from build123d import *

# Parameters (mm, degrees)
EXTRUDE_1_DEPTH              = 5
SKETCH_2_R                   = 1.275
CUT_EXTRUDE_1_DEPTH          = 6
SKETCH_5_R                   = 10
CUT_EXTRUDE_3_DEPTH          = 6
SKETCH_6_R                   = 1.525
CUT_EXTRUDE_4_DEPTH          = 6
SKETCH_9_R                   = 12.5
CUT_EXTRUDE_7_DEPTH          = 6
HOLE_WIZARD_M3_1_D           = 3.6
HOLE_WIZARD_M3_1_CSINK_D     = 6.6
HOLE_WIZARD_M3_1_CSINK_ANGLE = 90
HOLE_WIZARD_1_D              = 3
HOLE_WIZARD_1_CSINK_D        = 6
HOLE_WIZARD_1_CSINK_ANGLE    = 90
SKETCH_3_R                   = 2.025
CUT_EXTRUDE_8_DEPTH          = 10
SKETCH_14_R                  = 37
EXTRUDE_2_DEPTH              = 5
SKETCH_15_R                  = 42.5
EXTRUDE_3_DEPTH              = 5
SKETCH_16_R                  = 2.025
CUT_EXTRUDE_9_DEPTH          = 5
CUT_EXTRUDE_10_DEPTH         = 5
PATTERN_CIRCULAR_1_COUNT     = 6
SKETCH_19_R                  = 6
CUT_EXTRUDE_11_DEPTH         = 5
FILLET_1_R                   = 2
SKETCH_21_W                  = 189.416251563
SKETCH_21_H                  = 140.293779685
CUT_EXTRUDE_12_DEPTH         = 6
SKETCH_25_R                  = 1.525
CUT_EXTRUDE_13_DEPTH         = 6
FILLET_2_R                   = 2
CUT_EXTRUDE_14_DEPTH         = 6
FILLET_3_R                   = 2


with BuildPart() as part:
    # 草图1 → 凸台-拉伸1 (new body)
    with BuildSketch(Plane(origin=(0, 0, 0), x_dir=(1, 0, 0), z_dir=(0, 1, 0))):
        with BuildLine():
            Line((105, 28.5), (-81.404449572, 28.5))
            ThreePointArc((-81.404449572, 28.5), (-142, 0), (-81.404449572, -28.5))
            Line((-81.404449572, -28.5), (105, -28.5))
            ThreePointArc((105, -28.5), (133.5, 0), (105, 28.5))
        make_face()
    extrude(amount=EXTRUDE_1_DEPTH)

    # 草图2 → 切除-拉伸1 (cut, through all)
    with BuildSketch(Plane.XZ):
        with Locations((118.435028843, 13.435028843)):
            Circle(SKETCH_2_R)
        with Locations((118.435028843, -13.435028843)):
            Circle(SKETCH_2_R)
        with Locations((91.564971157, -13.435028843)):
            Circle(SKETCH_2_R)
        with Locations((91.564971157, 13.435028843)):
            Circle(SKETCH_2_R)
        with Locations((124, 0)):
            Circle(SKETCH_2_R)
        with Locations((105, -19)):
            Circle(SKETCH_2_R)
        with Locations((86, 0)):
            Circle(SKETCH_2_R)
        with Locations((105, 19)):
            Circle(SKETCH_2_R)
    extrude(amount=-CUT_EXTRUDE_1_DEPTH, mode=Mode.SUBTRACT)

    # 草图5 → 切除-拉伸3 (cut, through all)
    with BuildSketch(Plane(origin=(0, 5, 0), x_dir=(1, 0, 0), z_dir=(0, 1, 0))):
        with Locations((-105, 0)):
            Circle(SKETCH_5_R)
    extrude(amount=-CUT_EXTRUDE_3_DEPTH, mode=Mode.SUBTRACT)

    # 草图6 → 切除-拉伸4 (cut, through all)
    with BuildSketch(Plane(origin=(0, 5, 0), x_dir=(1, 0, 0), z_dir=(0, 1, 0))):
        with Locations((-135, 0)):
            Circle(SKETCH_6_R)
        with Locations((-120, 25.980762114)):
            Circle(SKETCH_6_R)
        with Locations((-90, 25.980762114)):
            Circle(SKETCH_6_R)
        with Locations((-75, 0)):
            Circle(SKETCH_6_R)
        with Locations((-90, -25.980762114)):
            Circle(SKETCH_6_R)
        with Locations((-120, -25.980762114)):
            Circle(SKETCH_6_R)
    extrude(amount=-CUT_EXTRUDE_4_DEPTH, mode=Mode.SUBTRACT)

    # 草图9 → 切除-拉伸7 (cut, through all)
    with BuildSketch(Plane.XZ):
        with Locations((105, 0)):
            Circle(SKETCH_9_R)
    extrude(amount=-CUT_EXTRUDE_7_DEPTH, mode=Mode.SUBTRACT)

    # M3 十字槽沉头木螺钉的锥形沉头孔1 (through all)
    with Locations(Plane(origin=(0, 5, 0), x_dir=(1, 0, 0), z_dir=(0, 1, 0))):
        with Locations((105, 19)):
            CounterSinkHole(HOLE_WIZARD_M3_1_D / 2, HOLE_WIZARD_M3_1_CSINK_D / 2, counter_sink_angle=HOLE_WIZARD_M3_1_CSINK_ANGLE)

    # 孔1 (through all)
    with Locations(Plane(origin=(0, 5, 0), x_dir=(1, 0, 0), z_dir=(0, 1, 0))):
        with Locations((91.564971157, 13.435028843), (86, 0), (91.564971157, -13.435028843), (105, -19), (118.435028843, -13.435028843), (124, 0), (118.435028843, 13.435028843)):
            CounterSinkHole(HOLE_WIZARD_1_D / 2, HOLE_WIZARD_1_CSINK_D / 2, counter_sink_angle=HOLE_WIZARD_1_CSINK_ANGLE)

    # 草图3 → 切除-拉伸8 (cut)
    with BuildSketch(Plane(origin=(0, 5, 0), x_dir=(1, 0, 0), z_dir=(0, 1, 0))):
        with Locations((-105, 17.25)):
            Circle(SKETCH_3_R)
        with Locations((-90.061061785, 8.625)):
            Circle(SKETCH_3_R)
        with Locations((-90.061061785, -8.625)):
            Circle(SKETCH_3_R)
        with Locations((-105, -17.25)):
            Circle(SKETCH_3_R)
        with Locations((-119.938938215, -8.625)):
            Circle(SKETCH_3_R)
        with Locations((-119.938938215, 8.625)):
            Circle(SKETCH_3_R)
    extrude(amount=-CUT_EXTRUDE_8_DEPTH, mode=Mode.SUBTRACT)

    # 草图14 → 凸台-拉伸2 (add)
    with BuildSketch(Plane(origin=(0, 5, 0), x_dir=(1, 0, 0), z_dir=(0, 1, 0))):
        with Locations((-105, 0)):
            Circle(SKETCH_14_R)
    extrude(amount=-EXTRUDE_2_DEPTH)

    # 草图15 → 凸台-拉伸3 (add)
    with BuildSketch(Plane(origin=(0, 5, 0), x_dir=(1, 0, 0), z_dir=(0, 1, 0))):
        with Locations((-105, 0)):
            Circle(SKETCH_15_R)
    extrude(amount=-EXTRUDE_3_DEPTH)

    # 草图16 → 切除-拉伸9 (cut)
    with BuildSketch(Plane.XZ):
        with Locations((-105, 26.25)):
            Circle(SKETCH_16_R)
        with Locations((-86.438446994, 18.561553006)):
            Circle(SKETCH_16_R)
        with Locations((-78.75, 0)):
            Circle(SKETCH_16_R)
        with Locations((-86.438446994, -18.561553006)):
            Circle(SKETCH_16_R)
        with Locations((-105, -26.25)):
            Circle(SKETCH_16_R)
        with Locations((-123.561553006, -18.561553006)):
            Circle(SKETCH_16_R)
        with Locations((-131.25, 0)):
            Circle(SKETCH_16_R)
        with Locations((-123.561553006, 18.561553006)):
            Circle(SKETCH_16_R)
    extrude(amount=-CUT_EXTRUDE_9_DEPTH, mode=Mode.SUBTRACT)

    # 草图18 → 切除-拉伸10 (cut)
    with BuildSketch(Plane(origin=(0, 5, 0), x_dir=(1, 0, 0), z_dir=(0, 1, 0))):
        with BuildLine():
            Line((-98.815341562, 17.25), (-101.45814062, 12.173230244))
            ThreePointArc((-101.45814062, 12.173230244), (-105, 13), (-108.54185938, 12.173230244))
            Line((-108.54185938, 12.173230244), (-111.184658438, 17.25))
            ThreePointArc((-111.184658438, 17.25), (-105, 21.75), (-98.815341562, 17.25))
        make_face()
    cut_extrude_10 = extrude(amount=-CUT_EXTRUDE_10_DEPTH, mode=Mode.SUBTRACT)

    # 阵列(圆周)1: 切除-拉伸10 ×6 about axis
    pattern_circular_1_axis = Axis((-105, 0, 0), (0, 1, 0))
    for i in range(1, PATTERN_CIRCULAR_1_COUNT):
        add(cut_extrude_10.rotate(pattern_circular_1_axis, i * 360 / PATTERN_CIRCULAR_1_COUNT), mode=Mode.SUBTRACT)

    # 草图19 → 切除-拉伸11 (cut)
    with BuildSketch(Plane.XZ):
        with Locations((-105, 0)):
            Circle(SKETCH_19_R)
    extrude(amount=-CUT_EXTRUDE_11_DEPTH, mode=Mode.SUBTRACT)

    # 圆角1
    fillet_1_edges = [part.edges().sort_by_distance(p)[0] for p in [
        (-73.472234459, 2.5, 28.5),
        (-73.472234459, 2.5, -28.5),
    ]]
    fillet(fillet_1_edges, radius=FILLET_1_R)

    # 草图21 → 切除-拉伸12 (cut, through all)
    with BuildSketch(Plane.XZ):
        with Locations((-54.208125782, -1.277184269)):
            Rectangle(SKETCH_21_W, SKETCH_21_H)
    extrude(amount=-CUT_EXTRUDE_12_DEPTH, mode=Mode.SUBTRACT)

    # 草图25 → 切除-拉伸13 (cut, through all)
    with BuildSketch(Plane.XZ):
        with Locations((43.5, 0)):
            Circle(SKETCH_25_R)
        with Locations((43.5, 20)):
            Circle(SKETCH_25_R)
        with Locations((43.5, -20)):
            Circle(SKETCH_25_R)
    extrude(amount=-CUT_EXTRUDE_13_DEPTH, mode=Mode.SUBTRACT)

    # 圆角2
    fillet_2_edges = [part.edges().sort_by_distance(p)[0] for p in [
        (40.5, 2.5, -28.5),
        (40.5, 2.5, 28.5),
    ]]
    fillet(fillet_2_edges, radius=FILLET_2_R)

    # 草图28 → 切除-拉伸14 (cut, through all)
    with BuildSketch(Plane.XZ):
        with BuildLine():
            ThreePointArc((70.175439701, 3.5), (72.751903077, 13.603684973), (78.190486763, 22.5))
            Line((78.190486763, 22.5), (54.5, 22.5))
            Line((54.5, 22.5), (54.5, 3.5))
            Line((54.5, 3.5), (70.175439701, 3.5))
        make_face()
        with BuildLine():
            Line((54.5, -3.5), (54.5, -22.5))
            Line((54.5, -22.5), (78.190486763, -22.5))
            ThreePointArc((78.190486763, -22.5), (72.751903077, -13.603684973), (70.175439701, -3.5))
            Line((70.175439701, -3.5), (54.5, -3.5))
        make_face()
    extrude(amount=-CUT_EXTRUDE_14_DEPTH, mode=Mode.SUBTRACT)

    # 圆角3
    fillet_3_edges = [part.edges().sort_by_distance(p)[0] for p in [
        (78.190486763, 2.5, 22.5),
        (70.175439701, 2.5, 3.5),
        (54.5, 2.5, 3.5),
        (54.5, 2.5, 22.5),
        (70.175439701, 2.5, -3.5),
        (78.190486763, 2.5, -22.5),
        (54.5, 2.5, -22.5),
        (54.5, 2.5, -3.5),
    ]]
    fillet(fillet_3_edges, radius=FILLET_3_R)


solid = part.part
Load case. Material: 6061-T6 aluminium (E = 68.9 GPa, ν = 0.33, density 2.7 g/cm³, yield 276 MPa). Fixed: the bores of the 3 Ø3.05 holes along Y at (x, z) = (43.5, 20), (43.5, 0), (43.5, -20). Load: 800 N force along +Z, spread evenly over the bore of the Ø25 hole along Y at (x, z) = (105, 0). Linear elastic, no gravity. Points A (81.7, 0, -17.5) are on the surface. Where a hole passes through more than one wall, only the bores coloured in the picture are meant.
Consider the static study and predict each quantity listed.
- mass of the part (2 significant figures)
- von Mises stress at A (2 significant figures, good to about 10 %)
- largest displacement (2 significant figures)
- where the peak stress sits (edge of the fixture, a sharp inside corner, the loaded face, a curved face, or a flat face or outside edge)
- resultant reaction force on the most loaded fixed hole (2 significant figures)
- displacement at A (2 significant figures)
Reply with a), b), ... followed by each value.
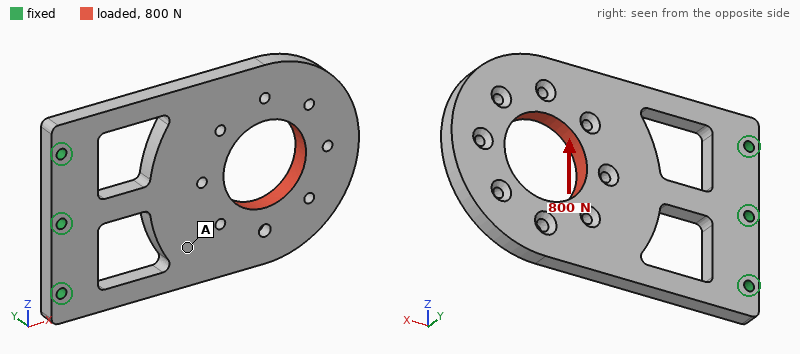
a) 49 g
b) 11 MPa
c) 0.10 mm
d) a curved face
e) 1.1 kN
f) 0.060 mm
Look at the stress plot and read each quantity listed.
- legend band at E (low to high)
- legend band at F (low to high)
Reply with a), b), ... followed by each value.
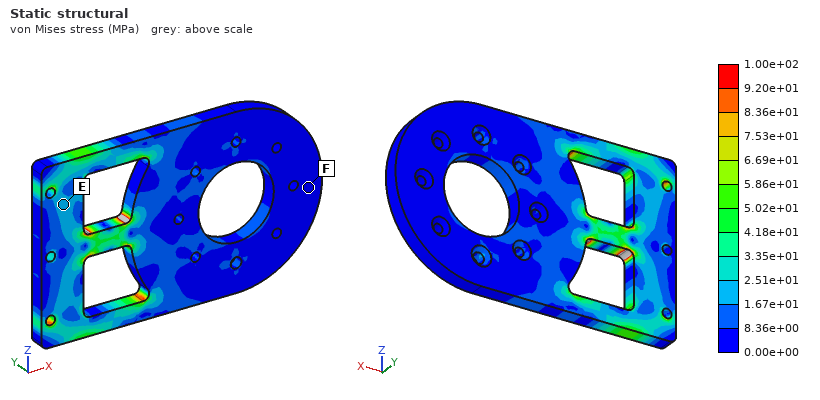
a) 1.67e+01 to 2.51e+01 MPa
b) 0.00e+00 to 8.36e+00 MPa
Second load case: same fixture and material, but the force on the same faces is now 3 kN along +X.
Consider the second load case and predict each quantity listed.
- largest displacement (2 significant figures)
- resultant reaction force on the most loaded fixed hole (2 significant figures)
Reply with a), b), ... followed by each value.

a) 29 µm
b) 1.0 kN
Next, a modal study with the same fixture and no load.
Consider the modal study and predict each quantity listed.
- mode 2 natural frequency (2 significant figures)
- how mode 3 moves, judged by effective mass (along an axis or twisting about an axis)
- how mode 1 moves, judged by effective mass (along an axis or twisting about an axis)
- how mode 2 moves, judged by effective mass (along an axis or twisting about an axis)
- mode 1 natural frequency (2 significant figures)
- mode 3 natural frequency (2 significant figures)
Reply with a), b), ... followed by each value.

a) 1600 Hz
b) along Z
c) along Y
d) twisting about X
e) 430 Hz
f) 2800 Hz
